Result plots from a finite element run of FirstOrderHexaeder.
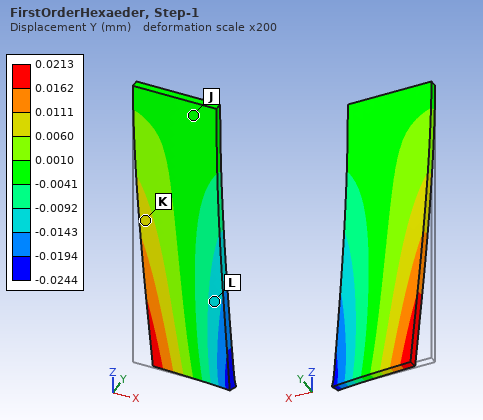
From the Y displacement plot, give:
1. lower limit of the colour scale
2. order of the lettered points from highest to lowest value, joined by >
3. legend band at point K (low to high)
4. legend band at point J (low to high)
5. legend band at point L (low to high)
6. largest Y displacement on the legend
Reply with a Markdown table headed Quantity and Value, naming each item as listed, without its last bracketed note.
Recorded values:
| Quantity | Value |
|---|---|
| lower limit of the colour scale | -0.0244 mm |
| order of the lettered points from highest to lowest value, joined by > | K > J > L |
| legend band at point K | 0.0060 to 0.0111 mm |
| legend band at point J | -0.0041 to 0.0010 mm |
| legend band at point L | -0.0143 to -0.0092 mm |
| largest Y displacement on the legend | 0.0213 mm |
